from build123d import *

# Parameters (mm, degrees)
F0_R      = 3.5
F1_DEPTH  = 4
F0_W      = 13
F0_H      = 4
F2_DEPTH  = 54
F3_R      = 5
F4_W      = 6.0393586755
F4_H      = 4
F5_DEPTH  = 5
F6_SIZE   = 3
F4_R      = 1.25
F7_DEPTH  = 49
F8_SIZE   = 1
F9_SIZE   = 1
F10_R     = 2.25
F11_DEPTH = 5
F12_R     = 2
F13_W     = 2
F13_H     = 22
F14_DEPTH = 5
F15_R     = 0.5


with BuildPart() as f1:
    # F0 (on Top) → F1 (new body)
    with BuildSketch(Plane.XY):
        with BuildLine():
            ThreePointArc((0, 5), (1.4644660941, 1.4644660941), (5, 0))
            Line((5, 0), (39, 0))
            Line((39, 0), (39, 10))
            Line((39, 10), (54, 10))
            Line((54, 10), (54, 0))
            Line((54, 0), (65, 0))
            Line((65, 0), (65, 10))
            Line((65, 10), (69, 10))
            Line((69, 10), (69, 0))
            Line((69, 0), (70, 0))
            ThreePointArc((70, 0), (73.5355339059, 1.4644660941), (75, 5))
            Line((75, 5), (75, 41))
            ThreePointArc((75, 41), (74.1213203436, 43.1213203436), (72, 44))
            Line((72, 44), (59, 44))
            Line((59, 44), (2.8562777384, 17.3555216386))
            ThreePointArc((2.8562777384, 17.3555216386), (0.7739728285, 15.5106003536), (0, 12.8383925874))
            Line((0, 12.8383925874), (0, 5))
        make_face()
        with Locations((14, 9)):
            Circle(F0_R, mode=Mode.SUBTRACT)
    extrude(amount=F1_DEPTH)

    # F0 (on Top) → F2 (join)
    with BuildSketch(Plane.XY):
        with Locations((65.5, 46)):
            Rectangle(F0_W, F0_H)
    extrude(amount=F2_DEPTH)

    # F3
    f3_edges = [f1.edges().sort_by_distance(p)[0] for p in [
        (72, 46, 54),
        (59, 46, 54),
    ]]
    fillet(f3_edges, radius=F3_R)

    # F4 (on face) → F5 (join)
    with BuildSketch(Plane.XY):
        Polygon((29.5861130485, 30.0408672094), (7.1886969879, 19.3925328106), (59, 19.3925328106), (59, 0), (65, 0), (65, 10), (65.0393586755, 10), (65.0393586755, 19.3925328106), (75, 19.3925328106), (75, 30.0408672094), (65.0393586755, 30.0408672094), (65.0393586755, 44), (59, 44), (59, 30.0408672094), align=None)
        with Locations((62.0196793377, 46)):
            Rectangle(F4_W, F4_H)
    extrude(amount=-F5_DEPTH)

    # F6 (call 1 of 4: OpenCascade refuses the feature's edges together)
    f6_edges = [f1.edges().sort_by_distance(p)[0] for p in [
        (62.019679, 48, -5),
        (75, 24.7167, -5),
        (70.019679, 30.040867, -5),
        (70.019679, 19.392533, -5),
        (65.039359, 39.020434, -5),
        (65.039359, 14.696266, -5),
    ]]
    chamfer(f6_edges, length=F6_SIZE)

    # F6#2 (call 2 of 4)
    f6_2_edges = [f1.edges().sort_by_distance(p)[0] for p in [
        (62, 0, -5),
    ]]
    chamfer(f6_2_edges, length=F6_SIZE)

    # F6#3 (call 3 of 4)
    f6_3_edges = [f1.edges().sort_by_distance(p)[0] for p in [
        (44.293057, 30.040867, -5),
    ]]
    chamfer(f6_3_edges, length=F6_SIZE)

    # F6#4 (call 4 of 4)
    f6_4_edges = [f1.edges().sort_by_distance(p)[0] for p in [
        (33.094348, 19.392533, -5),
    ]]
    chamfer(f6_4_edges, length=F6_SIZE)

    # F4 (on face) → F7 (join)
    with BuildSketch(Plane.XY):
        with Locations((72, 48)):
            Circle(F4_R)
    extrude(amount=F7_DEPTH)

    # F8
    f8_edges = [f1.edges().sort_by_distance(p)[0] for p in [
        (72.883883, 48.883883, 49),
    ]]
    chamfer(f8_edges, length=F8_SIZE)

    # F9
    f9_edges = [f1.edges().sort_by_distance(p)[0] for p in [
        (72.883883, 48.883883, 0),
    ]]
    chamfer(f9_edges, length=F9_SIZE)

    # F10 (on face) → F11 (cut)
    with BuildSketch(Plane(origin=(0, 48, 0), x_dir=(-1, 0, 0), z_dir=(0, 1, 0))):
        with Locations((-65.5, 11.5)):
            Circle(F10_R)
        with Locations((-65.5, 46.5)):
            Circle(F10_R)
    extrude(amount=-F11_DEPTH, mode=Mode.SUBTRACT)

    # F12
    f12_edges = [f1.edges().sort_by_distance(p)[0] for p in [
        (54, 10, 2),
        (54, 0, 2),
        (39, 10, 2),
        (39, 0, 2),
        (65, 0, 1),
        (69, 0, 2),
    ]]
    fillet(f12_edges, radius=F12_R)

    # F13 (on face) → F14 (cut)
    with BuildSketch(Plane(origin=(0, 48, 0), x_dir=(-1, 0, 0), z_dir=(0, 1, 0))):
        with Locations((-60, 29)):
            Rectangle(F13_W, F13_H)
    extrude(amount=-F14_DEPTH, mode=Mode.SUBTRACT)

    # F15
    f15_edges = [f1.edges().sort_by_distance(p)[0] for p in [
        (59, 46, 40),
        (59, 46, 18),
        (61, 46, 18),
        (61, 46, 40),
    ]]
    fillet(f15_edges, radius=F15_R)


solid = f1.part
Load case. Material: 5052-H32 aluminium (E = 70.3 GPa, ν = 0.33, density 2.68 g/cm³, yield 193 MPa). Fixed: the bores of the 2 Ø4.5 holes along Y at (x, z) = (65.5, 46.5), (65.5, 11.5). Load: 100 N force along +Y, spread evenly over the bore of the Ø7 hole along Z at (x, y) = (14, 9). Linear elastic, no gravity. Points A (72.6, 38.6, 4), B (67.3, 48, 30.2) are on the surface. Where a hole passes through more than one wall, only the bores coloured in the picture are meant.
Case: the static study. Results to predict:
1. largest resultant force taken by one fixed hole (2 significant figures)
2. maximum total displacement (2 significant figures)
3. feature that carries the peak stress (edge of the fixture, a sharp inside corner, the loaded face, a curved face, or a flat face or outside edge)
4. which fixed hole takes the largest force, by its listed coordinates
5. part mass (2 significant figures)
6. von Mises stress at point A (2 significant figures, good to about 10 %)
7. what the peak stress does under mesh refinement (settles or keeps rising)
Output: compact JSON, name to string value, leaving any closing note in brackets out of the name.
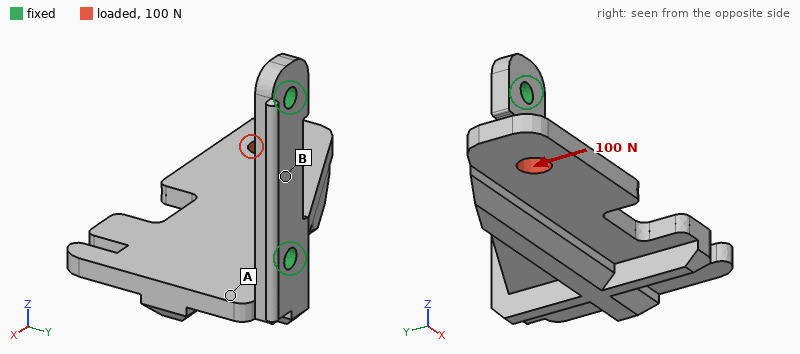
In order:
{"largest resultant force taken by one fixed hole": "97 N", "maximum total displacement": "0.44 mm", "feature that carries the peak stress": "edge of the fixture", "which fixed hole takes the largest force, by its listed coordinates": "(65.5, 11.5)", "part mass": "40 g", "von Mises stress at point A": "19 MPa", "what the peak stress does under mesh refinement": "keeps rising"}
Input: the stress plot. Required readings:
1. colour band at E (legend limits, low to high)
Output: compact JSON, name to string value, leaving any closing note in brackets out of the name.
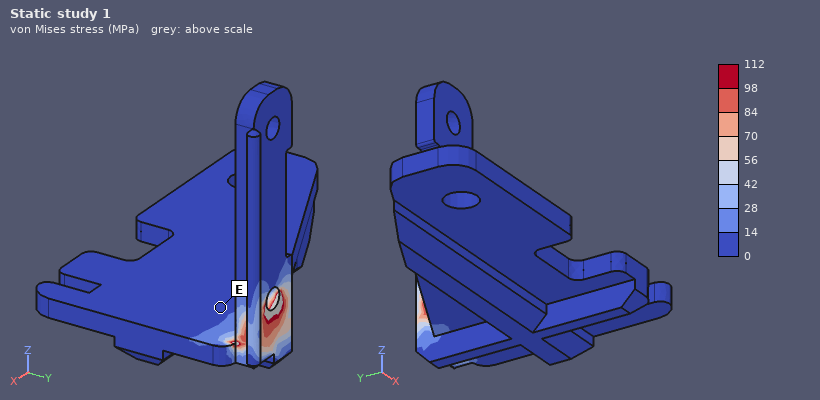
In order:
{"colour band at E": "0 to 14 MPa"}
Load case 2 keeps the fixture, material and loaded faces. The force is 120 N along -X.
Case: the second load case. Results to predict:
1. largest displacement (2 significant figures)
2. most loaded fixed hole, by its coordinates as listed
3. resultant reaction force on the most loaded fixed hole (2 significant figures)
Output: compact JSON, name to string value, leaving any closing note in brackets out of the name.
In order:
{"largest displacement": "0.36 mm", "most loaded fixed hole, by its coordinates as listed": "(65.5, 11.5)", "resultant reaction force on the most loaded fixed hole": "140 N"}
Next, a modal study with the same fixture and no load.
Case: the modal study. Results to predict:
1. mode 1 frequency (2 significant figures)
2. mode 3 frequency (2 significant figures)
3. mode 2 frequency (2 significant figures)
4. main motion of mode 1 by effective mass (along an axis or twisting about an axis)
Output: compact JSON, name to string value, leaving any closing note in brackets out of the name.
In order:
{"mode 1 frequency": "570 Hz", "mode 3 frequency": "1600 Hz", "mode 2 frequency": "720 Hz", "main motion of mode 1 by effective mass": "along Z"}
